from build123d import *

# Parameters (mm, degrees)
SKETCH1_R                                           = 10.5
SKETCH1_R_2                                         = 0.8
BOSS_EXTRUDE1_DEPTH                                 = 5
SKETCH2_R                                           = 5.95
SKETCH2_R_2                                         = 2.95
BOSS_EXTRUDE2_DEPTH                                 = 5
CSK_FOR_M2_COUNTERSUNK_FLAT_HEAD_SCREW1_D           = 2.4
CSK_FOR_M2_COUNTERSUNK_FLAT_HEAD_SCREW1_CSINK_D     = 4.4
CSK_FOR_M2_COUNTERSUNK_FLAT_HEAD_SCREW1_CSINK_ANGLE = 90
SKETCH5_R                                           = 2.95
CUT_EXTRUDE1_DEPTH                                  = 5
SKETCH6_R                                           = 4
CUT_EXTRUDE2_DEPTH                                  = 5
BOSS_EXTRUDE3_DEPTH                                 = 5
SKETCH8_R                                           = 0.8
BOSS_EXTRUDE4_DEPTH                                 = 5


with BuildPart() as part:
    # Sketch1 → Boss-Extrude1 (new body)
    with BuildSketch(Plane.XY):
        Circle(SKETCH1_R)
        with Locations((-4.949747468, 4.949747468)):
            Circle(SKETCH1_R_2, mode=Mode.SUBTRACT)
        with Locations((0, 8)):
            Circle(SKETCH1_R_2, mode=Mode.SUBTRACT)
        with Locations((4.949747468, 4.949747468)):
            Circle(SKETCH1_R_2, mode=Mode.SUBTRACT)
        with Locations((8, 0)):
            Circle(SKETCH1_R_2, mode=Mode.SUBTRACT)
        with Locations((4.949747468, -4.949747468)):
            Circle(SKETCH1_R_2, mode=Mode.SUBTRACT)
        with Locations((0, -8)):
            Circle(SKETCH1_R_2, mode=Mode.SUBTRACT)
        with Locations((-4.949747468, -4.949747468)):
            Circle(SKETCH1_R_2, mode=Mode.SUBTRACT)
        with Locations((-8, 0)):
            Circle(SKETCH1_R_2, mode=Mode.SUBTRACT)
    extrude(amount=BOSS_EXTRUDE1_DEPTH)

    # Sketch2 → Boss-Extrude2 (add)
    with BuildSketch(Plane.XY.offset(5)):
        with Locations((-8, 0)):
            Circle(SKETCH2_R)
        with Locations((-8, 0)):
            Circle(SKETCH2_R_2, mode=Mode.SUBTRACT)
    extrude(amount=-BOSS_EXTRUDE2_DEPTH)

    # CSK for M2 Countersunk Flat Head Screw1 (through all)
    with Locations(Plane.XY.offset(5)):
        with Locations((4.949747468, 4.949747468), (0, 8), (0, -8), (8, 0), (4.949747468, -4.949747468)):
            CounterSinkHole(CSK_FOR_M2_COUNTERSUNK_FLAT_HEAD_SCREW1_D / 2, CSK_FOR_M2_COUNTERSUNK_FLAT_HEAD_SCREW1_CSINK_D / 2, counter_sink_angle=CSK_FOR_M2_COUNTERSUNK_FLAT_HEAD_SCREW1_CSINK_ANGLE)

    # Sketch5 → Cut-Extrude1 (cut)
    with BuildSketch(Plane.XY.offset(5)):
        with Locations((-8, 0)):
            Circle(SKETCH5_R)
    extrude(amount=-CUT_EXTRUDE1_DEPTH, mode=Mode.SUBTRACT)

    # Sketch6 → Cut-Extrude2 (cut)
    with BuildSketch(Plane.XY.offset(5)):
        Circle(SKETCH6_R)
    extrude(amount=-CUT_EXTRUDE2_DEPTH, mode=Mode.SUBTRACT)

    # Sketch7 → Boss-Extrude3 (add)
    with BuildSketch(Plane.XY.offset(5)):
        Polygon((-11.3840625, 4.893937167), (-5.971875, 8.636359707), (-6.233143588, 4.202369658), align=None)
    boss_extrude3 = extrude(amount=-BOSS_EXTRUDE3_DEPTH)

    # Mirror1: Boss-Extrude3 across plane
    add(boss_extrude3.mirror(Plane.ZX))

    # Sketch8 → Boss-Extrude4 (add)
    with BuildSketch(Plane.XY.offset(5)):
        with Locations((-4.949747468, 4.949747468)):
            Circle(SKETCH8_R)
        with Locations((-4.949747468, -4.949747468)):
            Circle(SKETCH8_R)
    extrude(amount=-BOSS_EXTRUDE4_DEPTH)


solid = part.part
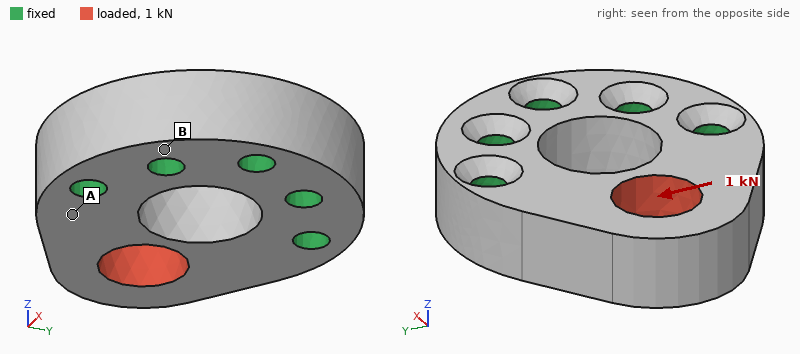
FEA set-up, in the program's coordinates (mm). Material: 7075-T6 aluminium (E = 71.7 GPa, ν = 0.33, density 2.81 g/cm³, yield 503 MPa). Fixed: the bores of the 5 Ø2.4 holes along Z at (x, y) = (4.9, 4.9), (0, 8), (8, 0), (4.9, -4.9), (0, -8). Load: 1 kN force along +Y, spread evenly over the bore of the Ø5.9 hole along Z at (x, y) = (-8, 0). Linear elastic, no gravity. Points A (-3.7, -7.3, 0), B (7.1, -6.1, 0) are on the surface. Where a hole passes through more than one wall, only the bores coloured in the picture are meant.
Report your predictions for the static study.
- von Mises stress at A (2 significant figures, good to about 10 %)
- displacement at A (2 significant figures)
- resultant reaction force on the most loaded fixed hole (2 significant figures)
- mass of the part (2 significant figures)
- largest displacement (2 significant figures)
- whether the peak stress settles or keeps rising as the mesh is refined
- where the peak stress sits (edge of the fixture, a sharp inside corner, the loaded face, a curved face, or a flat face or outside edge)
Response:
30 MPa
3.5 µm
700 N
3.9 g
13 µm
keeps rising
edge of the fixture
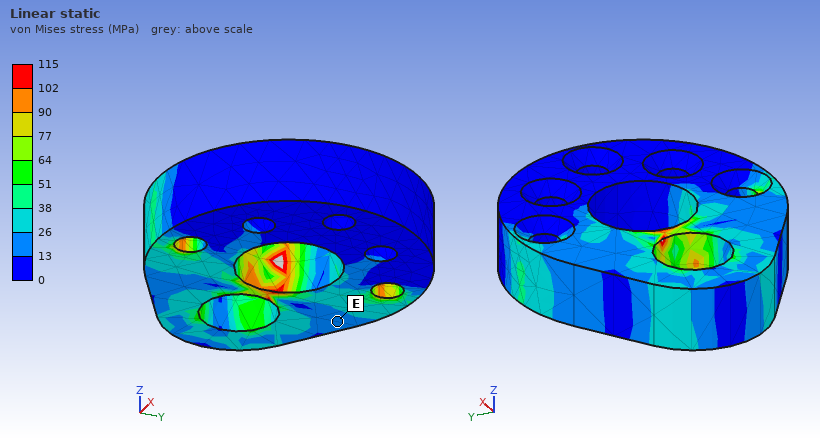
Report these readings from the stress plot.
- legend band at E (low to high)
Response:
13 to 26 MPa
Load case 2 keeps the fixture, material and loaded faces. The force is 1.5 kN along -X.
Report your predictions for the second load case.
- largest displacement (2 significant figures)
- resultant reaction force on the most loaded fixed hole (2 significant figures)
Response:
7.4 µm
660 N
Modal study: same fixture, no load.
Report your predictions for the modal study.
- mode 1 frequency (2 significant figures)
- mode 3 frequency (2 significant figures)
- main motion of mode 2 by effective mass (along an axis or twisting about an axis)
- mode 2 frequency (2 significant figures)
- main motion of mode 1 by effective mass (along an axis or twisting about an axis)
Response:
21 kHz
49 kHz
along Y
42 kHz
along Z
